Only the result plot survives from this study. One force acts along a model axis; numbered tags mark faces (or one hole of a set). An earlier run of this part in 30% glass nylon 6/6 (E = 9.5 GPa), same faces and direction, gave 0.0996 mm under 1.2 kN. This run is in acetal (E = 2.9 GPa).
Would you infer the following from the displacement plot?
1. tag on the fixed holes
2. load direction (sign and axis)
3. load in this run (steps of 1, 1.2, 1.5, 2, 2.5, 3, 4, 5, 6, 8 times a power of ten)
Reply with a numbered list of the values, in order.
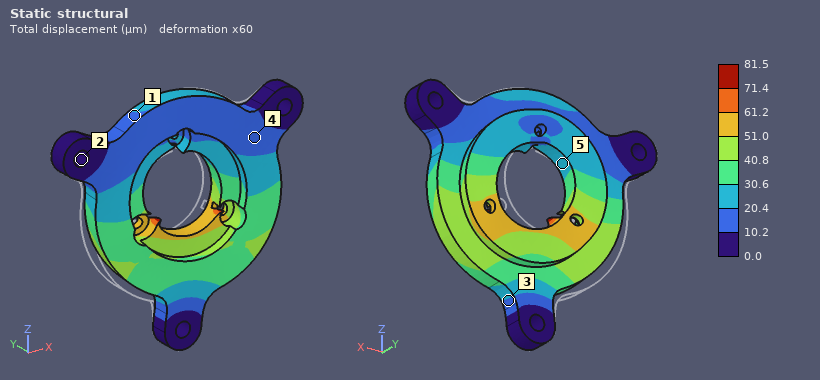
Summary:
1. 2
2. +X
3. 300 N
